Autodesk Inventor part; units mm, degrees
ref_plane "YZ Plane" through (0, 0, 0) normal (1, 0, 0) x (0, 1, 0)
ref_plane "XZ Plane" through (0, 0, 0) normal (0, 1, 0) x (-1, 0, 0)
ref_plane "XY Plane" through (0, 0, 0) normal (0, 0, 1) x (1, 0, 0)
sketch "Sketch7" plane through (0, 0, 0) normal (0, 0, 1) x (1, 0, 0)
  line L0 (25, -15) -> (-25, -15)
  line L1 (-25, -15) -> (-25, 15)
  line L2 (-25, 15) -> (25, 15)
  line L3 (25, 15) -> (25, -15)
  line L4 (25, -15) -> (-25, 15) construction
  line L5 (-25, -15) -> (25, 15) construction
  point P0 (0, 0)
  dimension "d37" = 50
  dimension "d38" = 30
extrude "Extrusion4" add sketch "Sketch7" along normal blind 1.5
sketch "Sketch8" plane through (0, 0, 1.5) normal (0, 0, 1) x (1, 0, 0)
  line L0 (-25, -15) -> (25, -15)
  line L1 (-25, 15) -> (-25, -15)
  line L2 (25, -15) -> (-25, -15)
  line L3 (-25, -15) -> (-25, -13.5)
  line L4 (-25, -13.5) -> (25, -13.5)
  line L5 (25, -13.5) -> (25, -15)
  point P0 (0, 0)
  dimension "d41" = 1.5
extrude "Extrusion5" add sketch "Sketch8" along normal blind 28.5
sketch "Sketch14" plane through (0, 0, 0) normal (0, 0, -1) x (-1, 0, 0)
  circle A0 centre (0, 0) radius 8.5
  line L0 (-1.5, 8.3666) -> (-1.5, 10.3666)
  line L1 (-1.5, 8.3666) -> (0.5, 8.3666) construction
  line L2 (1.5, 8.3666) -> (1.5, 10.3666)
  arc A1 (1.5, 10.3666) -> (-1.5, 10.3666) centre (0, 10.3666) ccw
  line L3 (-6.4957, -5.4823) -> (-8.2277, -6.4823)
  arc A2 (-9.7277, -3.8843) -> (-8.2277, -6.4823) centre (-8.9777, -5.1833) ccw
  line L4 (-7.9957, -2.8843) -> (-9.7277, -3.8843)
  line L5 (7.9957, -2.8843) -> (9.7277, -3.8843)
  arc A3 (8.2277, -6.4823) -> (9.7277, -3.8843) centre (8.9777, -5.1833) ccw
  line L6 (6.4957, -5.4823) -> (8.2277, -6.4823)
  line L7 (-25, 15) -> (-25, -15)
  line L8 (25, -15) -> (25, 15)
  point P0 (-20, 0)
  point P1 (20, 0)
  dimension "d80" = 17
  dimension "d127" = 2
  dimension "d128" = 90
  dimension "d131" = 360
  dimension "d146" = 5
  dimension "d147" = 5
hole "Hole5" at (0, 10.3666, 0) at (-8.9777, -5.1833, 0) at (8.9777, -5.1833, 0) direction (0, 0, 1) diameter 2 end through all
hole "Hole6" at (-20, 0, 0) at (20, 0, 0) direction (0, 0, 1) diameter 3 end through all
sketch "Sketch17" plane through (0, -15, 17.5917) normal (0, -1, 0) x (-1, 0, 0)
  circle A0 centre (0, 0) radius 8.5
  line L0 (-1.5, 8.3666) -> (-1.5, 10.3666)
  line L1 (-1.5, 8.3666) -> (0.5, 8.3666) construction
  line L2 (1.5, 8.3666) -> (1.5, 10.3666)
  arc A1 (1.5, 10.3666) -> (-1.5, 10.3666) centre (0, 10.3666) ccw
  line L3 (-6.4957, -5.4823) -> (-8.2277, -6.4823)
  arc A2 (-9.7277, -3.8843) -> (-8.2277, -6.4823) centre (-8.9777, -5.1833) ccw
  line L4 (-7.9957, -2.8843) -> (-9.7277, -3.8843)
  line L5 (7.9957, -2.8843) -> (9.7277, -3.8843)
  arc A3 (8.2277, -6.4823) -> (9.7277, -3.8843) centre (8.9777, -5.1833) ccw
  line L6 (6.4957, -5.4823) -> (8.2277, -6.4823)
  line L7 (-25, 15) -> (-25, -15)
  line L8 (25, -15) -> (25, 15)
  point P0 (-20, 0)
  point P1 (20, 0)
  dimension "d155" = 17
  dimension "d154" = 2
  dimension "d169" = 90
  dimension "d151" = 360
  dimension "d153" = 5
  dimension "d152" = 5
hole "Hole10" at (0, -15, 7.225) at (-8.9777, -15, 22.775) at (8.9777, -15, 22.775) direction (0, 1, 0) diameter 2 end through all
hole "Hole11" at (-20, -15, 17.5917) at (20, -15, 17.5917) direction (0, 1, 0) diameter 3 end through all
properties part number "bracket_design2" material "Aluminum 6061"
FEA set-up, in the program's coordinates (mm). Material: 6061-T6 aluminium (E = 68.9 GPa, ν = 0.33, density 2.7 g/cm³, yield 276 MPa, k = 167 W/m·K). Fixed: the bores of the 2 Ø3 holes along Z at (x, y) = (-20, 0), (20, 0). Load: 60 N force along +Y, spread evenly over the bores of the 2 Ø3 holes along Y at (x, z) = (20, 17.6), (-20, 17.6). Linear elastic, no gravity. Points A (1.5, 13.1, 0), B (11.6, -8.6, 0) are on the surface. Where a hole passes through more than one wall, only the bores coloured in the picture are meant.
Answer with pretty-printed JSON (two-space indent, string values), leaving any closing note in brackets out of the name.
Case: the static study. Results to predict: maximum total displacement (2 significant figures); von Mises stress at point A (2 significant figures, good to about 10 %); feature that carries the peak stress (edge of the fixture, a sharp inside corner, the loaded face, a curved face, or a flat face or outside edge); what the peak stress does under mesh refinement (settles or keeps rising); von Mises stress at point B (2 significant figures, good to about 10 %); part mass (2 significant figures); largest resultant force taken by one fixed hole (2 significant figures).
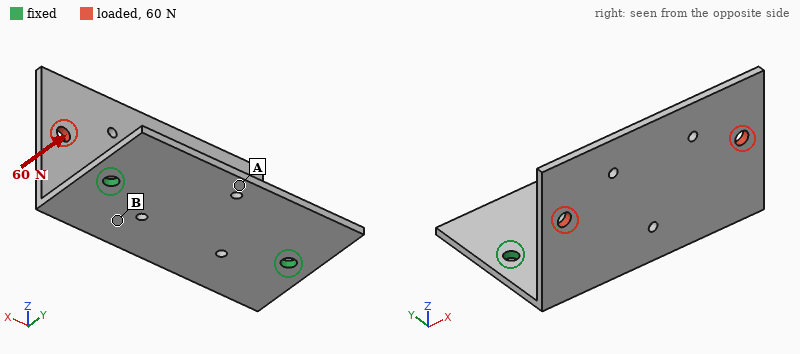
{
  "maximum total displacement": "0.67 mm",
  "von Mises stress at point A": "13 MPa",
  "feature that carries the peak stress": "edge of the fixture",
  "what the peak stress does under mesh refinement": "keeps rising",
  "von Mises stress at point B": "44 MPa",
  "part mass": "12 g",
  "largest resultant force taken by one fixed hole": "30 N"
}
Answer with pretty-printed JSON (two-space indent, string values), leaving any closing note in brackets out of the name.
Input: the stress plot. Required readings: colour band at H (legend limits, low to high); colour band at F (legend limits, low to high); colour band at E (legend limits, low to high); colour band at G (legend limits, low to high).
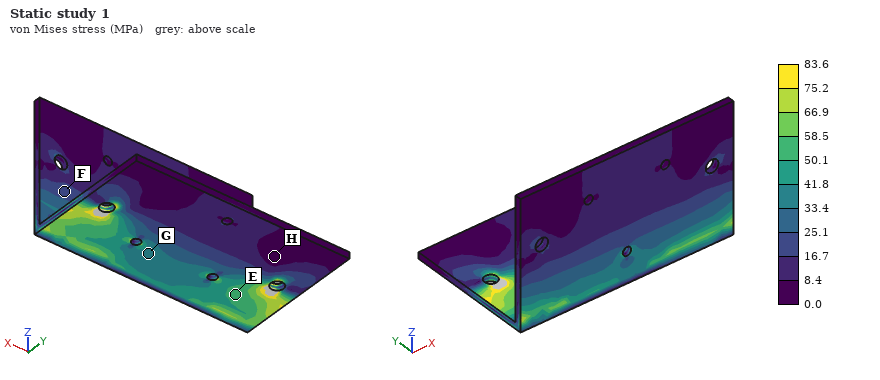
{
  "colour band at H": "0.0 to 8.4 MPa",
  "colour band at F": "16.7 to 25.1 MPa",
  "colour band at E": "50.1 to 58.5 MPa",
  "colour band at G": "33.4 to 41.8 MPa"
}
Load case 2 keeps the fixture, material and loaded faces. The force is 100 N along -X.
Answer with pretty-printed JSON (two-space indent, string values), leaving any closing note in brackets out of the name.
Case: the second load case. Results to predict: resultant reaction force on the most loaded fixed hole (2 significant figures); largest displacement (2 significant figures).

{
  "resultant reaction force on the most loaded fixed hole": "74 N",
  "largest displacement": "0.15 mm"
}
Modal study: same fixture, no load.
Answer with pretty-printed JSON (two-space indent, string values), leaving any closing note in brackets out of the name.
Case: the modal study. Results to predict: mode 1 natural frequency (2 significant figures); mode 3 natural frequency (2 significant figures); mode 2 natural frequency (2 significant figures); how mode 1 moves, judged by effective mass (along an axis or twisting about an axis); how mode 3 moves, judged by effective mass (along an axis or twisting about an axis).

{
  "mode 1 natural frequency": "790 Hz",
  "mode 3 natural frequency": "2500 Hz",
  "mode 2 natural frequency": "1700 Hz",
  "how mode 1 moves, judged by effective mass": "along Y",
  "how mode 3 moves, judged by effective mass": "along Z"
}
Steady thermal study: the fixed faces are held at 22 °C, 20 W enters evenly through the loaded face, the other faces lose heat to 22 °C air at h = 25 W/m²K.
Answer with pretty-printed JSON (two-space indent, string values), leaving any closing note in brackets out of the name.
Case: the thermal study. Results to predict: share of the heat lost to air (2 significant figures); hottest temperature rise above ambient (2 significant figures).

{
  "share of the heat lost to air": "21 %",
  "hottest temperature rise above ambient": "62 K"
}
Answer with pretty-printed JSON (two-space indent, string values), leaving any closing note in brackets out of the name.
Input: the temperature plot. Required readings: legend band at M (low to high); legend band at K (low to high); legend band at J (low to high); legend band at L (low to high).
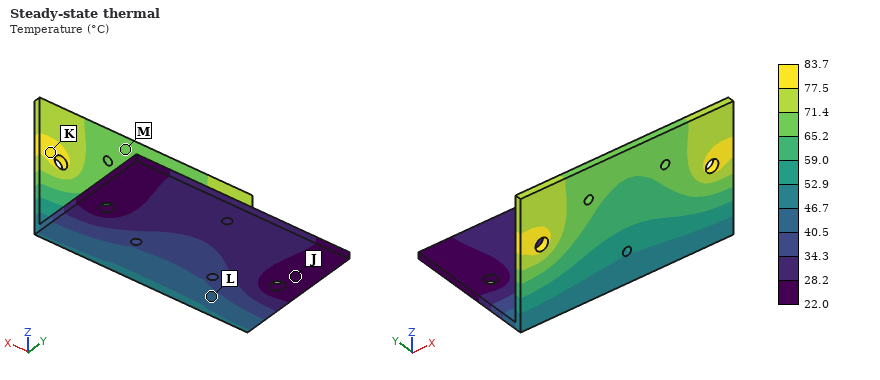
{
  "legend band at M": "65.2 to 71.4 °C",
  "legend band at K": "77.5 to 83.7 °C",
  "legend band at J": "22.0 to 28.2 °C",
  "legend band at L": "40.5 to 46.7 °C"
}
